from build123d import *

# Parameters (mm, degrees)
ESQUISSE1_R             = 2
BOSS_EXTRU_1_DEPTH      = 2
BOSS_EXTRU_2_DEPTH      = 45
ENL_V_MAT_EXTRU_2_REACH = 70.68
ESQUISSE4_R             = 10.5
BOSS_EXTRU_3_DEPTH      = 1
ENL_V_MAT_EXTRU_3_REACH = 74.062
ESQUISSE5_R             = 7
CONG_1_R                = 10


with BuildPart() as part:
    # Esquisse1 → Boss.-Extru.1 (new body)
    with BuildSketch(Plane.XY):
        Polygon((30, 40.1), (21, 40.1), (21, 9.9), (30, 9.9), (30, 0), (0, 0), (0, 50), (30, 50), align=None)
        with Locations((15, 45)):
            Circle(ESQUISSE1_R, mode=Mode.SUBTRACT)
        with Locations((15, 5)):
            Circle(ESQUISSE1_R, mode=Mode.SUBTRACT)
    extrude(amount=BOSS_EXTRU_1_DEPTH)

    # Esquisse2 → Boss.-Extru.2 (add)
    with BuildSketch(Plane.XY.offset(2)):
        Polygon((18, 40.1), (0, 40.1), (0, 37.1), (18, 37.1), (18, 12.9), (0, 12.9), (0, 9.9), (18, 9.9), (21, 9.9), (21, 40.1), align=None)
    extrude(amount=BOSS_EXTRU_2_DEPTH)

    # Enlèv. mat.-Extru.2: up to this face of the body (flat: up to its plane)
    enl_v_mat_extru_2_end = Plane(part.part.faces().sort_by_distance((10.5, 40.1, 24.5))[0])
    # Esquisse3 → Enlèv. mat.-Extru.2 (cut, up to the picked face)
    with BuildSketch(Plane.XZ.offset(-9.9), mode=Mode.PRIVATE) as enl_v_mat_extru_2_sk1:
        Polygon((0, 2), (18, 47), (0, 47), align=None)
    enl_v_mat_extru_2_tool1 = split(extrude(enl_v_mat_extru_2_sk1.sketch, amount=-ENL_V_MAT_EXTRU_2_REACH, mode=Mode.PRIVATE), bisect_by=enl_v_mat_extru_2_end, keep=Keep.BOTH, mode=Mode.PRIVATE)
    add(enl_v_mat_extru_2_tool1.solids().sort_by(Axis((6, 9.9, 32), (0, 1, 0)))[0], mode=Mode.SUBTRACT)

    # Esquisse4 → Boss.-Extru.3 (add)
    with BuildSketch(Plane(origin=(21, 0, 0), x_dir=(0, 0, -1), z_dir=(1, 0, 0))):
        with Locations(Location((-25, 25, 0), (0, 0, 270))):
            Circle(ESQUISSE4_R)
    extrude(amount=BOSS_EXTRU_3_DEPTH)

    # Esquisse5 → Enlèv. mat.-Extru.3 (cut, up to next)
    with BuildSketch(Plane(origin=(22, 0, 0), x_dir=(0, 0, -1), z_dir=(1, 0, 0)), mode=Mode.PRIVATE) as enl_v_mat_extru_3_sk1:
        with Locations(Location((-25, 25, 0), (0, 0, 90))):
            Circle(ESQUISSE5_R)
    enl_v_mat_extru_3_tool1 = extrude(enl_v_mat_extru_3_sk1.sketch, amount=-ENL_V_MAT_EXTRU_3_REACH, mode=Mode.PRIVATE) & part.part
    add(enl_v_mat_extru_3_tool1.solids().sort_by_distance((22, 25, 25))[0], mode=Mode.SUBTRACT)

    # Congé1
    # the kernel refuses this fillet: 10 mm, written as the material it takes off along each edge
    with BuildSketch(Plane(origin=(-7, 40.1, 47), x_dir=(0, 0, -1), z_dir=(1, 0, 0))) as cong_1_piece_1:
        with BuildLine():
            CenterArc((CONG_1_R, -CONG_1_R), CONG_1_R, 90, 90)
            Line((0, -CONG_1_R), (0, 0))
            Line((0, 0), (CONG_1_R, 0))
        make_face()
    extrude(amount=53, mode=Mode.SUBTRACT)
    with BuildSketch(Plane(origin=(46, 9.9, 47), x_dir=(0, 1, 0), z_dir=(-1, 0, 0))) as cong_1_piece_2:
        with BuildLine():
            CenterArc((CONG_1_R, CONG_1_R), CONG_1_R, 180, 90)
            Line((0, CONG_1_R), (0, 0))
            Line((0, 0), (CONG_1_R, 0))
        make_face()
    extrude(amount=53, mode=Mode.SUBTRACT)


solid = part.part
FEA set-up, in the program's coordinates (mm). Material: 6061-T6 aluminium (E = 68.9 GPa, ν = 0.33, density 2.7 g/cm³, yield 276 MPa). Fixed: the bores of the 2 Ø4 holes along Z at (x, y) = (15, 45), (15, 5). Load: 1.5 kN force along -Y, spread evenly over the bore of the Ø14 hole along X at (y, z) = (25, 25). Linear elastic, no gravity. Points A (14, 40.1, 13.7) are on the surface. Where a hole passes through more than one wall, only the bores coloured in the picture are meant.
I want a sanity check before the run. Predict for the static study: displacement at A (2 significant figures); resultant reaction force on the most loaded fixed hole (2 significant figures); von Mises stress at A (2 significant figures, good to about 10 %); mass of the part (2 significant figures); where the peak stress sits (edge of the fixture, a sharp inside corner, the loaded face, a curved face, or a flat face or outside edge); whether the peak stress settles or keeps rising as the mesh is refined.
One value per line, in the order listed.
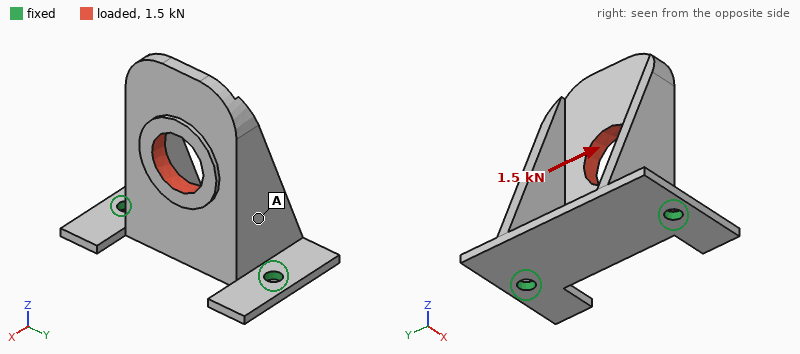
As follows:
0.055 mm
1.3 kN
27 MPa
23 g
edge of the fixture
keeps rising
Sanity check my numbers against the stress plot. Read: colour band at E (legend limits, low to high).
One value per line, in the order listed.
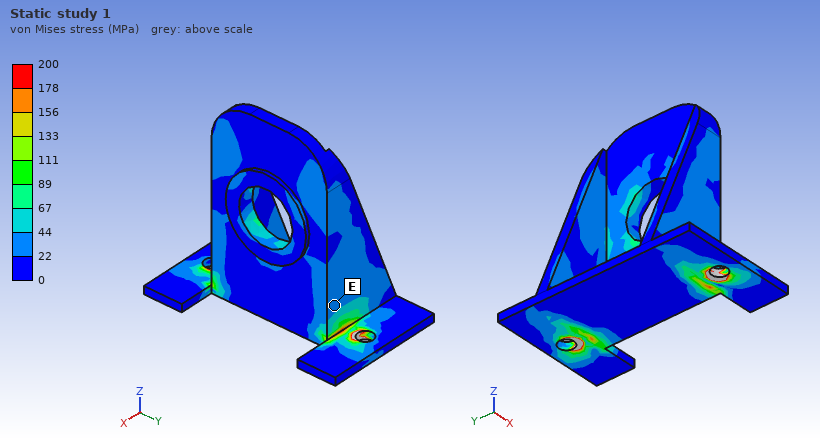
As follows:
22 to 44 MPa
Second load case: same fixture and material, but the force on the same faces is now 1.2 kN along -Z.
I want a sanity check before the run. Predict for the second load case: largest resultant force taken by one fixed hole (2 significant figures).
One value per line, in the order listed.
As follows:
680 N
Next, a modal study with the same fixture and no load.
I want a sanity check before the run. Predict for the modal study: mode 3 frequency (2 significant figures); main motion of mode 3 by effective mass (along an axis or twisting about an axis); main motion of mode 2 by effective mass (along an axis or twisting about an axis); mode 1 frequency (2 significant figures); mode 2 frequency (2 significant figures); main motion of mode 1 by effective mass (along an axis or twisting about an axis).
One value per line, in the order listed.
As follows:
6100 Hz
along Y
along Y
1400 Hz
3700 Hz
along X
